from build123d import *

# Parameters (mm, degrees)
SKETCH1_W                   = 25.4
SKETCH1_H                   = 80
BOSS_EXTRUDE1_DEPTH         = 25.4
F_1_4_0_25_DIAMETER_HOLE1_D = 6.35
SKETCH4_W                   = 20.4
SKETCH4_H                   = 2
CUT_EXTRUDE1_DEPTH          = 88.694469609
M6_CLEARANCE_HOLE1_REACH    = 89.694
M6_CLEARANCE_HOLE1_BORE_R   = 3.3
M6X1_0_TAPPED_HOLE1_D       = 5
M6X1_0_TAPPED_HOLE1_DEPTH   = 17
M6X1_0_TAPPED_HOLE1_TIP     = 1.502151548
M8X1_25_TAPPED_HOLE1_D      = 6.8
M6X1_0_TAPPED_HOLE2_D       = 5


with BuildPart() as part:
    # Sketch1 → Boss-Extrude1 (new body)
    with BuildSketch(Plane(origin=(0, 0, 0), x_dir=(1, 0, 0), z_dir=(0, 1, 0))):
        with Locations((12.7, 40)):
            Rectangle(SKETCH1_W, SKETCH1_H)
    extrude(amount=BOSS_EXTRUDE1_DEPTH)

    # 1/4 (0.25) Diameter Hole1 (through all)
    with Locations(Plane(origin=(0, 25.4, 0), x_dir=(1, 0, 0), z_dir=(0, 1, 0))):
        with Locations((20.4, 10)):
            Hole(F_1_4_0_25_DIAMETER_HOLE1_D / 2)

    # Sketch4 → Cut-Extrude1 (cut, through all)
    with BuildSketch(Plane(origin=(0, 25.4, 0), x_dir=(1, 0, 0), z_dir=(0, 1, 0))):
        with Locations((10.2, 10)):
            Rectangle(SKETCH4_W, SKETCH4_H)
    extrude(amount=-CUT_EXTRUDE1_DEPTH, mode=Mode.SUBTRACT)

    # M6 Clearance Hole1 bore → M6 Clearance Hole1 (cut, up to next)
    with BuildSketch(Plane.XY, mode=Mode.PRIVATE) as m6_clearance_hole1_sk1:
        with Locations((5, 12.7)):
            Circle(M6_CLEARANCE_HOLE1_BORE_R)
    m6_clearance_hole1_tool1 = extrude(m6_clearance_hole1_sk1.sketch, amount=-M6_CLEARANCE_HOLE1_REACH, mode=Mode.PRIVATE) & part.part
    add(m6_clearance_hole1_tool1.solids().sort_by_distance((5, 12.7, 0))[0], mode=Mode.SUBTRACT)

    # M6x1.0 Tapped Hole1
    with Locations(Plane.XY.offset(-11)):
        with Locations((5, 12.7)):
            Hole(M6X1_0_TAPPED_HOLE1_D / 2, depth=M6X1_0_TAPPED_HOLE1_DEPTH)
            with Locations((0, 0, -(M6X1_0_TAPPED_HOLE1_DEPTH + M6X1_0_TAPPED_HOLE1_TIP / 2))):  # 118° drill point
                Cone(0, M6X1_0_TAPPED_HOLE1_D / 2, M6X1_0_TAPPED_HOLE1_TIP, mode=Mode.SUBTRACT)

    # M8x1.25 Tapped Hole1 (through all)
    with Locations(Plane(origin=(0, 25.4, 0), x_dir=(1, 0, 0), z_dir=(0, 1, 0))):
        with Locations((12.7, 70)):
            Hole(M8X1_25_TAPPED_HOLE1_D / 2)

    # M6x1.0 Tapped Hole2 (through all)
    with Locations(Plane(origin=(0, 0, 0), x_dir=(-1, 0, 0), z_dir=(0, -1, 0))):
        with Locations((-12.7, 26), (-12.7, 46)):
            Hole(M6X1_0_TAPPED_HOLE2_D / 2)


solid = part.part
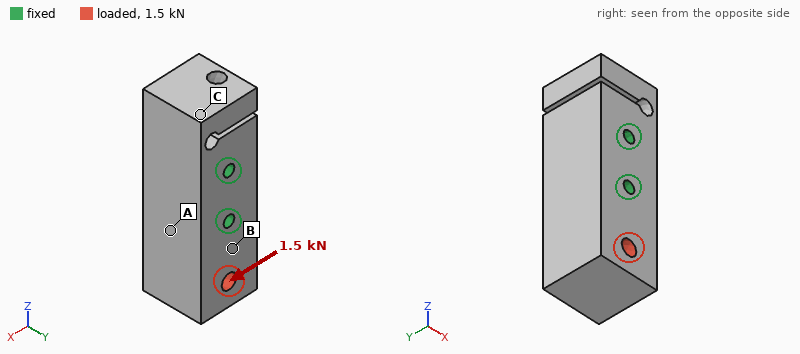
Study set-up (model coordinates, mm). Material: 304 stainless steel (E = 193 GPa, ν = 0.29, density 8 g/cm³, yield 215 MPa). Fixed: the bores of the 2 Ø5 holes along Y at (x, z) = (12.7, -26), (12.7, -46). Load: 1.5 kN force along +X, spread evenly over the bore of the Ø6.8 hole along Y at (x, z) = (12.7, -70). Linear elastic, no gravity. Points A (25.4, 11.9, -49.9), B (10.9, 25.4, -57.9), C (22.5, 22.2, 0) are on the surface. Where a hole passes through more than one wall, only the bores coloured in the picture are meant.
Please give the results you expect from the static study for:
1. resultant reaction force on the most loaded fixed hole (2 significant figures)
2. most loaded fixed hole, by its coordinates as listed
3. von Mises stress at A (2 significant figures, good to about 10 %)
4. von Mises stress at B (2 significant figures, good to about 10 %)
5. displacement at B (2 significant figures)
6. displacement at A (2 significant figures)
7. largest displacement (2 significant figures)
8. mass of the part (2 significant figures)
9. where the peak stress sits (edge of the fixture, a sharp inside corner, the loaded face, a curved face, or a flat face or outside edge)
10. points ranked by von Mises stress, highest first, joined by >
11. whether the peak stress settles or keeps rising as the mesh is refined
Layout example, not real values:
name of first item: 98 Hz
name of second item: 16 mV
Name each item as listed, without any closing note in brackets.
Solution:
resultant reaction force on the most loaded fixed hole: 2.7 kN
most loaded fixed hole, by its coordinates as listed: (12.7, -46)
von Mises stress at A: 11 MPa
von Mises stress at B: 6.4 MPa
displacement at B: 1.4 µm
displacement at A: 1.2 µm
largest displacement: 5.0 µm
mass of the part: 380 g
where the peak stress sits: edge of the fixture
points ranked by von Mises stress, highest first, joined by >: A > B > C
whether the peak stress settles or keeps rising as the mesh is refined: keeps rising
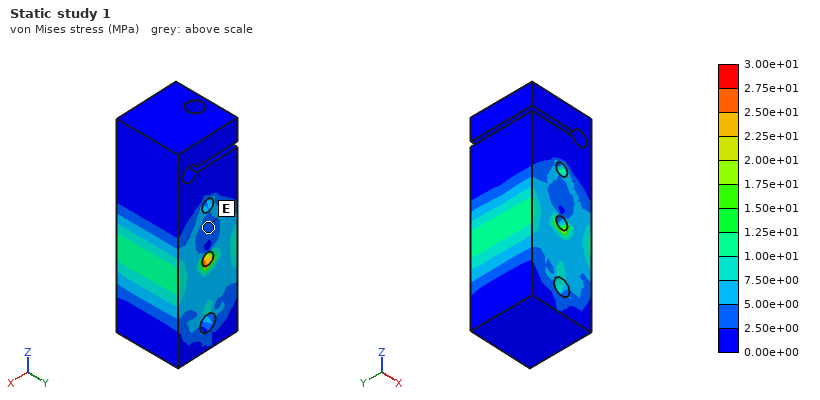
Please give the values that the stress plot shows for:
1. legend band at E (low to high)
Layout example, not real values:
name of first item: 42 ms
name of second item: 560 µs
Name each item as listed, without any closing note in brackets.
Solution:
legend band at E: 2.50e+00 to 5.00e+00 MPa
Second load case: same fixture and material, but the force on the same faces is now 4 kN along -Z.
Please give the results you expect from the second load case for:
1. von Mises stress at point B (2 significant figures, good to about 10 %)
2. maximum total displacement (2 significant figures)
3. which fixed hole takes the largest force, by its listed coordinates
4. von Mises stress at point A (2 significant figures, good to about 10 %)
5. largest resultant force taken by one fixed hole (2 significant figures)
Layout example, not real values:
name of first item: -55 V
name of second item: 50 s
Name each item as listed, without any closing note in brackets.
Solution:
von Mises stress at point B: 8.6 MPa
maximum total displacement: 1.4 µm
which fixed hole takes the largest force, by its listed coordinates: (12.7, -46)
von Mises stress at point A: 3.6 MPa
largest resultant force taken by one fixed hole: 3.2 kN
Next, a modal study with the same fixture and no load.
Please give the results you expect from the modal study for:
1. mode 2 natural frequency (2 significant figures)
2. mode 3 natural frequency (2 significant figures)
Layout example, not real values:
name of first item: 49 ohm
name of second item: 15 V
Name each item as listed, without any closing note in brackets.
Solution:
mode 2 natural frequency: 3800 Hz
mode 3 natural frequency: 8200 Hz
